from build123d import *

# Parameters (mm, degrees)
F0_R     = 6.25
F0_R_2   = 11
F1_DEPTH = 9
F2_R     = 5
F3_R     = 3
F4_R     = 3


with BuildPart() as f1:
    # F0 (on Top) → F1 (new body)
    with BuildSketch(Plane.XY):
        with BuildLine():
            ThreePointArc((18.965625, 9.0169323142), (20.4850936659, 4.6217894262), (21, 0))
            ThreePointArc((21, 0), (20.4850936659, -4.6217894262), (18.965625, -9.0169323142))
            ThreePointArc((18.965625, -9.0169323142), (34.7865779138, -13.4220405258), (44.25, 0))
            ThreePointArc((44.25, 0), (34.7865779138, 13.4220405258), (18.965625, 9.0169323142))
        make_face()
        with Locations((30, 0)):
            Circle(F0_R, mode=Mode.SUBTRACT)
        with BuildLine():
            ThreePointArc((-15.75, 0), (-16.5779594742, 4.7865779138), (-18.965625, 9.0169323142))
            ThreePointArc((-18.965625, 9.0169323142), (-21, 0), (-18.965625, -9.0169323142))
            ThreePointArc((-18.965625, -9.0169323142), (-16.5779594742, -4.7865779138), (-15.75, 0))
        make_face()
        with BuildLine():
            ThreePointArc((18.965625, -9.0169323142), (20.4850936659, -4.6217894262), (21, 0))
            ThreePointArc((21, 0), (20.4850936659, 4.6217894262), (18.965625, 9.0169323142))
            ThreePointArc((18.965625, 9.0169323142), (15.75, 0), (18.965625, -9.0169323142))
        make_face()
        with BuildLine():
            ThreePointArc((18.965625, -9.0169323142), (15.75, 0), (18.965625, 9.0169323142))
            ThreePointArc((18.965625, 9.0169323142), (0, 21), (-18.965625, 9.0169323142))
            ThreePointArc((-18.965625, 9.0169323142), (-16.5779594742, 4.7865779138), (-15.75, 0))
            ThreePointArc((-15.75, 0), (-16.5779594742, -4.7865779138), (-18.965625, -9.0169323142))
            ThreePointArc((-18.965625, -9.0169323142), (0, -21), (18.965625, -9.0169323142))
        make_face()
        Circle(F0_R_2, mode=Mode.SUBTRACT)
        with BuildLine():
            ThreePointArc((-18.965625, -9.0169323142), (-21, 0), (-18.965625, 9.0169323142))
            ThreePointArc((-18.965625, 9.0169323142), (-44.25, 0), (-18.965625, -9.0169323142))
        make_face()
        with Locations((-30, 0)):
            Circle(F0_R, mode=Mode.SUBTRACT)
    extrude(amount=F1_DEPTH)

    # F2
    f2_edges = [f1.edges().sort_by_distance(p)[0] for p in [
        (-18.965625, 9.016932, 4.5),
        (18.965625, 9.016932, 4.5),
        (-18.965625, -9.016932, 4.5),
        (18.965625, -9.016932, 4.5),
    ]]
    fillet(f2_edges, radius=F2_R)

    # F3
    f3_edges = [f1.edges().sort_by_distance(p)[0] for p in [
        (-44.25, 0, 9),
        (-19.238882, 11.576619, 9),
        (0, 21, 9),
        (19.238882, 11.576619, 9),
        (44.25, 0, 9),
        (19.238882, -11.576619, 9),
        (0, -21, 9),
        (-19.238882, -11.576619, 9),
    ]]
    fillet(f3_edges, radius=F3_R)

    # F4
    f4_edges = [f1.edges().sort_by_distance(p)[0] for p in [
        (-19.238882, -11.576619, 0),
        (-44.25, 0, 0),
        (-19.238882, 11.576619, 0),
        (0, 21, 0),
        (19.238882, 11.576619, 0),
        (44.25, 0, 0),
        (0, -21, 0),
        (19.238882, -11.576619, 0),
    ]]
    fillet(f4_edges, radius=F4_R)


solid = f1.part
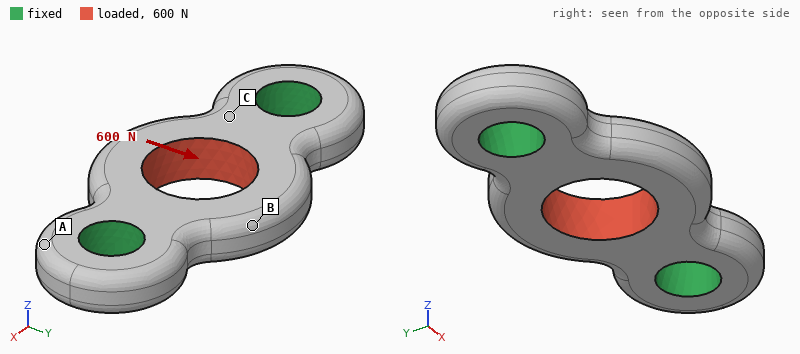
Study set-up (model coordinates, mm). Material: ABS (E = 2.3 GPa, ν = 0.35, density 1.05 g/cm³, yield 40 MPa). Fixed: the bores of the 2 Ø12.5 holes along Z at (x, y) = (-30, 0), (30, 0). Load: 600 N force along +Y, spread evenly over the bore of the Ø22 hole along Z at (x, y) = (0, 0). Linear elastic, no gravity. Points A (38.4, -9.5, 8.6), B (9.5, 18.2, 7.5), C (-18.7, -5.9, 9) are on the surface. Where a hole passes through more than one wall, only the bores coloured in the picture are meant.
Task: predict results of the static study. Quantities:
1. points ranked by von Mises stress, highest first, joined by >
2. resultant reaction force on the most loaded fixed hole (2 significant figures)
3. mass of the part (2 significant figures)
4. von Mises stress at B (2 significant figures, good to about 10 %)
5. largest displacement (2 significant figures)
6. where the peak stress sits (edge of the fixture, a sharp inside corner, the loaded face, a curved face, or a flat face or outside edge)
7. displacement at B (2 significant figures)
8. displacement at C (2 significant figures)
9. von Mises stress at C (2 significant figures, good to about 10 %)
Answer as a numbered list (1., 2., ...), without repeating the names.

1. C > B > A
2. 300 N
3. 17 g
4. 1.8 MPa
5. 42 µm
6. edge of the fixture
7. 34 µm
8. 16 µm
9. 2.8 MPa
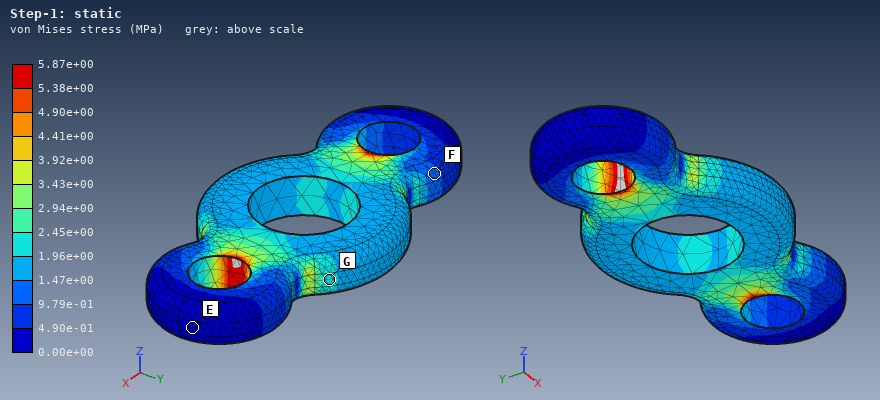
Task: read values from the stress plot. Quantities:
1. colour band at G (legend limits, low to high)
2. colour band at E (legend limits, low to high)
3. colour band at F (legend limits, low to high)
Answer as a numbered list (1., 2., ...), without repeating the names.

1. 1.96e+00 to 2.45e+00 MPa
2. 0.00e+00 to 4.90e-01 MPa
3. 9.79e-01 to 1.47e+00 MPa
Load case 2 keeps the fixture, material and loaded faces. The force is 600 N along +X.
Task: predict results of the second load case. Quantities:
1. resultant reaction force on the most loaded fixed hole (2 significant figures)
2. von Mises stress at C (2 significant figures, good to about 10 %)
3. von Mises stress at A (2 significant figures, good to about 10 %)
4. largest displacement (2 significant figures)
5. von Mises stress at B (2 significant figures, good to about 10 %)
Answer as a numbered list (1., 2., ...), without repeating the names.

1. 300 N
2. 1.4 MPa
3. 0.25 MPa
4. 19 µm
5. 0.56 MPa
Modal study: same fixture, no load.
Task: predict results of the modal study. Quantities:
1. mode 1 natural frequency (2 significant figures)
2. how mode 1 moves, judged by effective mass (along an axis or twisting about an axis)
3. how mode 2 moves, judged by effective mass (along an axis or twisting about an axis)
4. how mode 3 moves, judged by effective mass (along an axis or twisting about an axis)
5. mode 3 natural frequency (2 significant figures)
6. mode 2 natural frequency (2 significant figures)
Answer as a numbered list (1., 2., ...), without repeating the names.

1. 3400 Hz
2. twisting about X
3. along Z
4. along Y
5. 7500 Hz
6. 3700 Hz
